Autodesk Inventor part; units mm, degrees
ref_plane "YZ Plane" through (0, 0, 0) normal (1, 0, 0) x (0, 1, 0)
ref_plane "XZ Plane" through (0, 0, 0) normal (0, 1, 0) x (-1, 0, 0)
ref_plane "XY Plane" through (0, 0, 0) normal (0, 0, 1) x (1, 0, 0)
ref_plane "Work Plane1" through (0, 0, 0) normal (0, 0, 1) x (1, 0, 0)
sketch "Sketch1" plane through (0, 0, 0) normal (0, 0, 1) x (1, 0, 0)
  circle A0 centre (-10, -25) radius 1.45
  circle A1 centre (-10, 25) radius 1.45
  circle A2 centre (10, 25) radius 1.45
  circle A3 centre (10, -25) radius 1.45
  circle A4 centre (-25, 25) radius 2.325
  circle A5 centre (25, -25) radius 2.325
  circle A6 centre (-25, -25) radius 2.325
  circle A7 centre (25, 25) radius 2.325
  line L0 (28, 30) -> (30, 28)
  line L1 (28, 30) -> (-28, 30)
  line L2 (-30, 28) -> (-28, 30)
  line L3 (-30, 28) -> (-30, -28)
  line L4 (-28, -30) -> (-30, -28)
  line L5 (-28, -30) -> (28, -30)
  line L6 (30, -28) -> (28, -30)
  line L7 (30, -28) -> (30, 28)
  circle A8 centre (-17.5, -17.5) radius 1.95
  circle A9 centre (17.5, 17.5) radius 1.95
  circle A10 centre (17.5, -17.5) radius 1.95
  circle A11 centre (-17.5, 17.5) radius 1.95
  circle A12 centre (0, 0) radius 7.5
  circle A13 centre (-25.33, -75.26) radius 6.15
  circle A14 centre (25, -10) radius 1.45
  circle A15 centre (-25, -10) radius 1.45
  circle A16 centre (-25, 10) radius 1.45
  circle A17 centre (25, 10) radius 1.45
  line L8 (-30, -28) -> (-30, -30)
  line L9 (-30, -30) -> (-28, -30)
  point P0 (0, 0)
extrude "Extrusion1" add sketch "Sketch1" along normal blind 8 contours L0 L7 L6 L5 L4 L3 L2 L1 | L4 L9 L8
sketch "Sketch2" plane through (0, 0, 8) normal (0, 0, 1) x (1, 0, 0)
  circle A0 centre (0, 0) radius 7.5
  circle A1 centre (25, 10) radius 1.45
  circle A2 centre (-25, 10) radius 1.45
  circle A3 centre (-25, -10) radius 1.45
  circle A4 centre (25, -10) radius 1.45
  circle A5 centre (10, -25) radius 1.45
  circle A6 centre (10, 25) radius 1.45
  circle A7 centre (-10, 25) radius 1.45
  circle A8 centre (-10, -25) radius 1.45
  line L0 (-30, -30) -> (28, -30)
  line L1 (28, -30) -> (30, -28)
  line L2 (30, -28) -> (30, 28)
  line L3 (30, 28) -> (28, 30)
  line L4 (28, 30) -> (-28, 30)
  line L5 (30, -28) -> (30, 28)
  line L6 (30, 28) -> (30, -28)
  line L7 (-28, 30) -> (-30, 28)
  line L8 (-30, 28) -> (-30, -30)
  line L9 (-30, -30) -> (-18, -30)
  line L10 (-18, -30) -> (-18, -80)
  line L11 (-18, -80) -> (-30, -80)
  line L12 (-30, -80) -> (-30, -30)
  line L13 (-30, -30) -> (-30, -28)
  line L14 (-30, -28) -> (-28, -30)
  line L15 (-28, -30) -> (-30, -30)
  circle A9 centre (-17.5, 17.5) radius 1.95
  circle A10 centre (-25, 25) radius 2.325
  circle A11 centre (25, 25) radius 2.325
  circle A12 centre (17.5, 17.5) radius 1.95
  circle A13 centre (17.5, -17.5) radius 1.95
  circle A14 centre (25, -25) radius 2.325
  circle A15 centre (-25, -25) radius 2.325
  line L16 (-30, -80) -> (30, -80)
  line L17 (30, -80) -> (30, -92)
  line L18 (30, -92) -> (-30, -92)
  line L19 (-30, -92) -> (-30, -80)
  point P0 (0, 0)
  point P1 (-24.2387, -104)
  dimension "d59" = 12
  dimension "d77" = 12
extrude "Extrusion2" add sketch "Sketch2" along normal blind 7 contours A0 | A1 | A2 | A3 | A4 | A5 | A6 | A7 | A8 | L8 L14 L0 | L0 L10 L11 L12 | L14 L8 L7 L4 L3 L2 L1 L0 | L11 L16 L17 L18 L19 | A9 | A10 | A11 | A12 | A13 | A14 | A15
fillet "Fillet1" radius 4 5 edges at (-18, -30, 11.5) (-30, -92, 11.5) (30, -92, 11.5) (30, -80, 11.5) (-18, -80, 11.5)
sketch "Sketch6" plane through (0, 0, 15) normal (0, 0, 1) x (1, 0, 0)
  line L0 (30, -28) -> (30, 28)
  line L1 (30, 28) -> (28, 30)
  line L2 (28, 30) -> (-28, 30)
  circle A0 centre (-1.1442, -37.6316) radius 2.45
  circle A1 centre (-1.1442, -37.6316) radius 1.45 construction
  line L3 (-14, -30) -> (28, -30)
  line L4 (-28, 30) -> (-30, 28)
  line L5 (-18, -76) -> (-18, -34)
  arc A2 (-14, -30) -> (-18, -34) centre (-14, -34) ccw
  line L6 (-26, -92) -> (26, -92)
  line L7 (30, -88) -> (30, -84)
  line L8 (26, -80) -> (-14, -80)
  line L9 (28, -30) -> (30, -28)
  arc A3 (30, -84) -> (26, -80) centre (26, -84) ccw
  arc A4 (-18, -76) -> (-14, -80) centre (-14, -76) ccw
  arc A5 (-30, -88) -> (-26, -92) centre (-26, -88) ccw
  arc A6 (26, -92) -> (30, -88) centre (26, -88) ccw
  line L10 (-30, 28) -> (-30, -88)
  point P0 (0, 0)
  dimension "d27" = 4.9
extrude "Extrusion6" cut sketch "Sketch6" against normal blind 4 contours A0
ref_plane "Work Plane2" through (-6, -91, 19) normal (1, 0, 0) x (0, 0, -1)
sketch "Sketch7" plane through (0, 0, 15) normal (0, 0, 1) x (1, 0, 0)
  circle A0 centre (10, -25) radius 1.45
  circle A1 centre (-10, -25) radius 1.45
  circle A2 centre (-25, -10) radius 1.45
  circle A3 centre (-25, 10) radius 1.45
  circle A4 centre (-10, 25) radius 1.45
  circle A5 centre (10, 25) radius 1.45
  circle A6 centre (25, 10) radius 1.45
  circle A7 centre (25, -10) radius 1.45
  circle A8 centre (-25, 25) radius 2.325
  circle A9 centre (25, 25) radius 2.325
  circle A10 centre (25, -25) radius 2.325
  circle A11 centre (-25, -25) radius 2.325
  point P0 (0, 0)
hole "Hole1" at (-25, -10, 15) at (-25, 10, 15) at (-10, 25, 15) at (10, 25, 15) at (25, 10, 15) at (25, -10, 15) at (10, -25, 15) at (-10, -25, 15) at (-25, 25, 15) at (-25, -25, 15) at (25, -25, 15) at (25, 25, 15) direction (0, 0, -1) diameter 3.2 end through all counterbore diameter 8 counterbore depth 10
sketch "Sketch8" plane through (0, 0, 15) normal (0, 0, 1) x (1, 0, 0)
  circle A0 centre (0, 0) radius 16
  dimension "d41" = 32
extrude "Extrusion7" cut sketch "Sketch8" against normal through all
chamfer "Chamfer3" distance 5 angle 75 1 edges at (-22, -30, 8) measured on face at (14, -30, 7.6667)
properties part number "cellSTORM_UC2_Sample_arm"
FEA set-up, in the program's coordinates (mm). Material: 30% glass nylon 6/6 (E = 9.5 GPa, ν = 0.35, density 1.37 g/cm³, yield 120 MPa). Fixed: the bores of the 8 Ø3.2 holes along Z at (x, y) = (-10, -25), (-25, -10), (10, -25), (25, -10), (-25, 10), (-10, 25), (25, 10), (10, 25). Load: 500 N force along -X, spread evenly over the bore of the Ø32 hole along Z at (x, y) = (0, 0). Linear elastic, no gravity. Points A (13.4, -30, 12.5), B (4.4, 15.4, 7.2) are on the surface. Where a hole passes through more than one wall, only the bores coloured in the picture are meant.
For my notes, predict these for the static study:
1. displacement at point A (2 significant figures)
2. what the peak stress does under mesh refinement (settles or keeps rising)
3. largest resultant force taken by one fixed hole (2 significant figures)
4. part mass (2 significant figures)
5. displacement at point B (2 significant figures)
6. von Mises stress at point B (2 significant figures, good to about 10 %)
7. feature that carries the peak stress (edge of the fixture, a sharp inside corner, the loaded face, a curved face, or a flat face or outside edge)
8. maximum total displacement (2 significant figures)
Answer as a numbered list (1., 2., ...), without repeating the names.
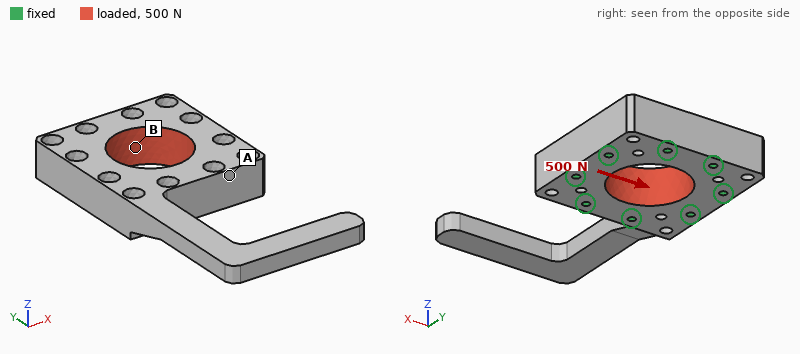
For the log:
1. 1.0 µm
2. keeps rising
3. 72 N
4. 61 g
5. 1.5 µm
6. 0.87 MPa
7. edge of the fixture
8. 4.8 µm
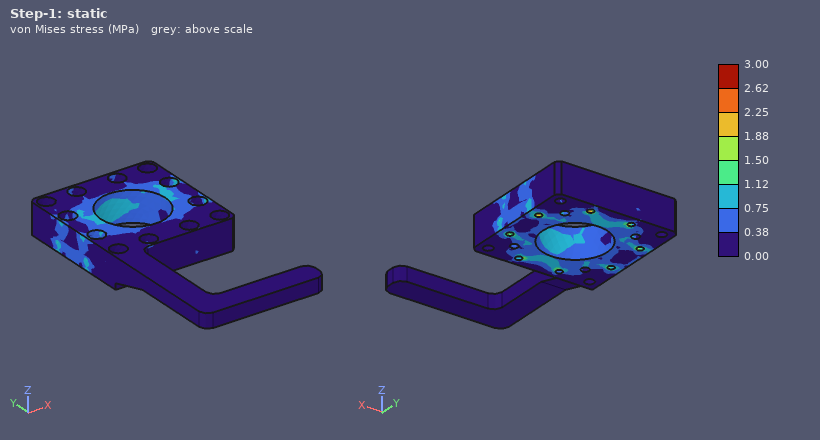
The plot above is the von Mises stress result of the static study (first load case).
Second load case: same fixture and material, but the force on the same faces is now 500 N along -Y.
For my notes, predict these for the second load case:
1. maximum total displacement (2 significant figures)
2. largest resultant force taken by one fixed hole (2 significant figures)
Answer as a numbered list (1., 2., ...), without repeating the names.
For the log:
1. 7.9 µm
2. 72 N
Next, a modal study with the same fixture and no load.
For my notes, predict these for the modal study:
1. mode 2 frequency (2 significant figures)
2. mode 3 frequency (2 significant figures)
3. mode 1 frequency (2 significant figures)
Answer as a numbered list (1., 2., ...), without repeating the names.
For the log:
1. 550 Hz
2. 950 Hz
3. 370 Hz
